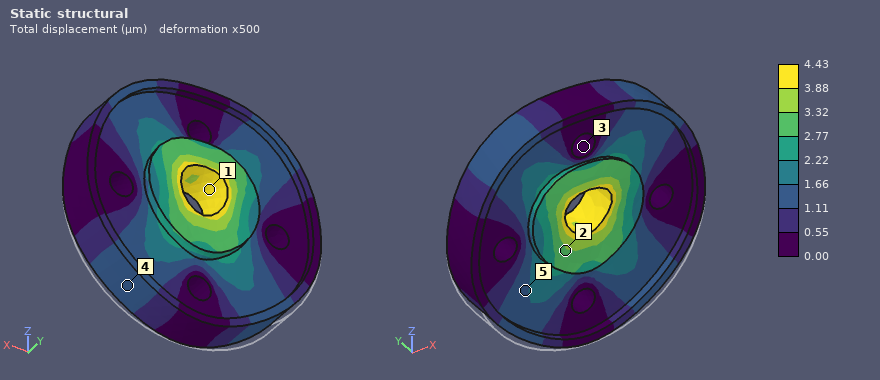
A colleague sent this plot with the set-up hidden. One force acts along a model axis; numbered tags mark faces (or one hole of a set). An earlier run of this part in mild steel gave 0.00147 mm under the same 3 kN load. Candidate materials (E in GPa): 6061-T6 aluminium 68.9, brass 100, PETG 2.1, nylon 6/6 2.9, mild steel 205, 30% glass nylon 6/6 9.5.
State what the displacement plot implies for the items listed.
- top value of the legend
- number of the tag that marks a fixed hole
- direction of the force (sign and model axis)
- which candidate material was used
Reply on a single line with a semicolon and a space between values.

4.43 µm; 3; +Z; 6061-T6 aluminium
